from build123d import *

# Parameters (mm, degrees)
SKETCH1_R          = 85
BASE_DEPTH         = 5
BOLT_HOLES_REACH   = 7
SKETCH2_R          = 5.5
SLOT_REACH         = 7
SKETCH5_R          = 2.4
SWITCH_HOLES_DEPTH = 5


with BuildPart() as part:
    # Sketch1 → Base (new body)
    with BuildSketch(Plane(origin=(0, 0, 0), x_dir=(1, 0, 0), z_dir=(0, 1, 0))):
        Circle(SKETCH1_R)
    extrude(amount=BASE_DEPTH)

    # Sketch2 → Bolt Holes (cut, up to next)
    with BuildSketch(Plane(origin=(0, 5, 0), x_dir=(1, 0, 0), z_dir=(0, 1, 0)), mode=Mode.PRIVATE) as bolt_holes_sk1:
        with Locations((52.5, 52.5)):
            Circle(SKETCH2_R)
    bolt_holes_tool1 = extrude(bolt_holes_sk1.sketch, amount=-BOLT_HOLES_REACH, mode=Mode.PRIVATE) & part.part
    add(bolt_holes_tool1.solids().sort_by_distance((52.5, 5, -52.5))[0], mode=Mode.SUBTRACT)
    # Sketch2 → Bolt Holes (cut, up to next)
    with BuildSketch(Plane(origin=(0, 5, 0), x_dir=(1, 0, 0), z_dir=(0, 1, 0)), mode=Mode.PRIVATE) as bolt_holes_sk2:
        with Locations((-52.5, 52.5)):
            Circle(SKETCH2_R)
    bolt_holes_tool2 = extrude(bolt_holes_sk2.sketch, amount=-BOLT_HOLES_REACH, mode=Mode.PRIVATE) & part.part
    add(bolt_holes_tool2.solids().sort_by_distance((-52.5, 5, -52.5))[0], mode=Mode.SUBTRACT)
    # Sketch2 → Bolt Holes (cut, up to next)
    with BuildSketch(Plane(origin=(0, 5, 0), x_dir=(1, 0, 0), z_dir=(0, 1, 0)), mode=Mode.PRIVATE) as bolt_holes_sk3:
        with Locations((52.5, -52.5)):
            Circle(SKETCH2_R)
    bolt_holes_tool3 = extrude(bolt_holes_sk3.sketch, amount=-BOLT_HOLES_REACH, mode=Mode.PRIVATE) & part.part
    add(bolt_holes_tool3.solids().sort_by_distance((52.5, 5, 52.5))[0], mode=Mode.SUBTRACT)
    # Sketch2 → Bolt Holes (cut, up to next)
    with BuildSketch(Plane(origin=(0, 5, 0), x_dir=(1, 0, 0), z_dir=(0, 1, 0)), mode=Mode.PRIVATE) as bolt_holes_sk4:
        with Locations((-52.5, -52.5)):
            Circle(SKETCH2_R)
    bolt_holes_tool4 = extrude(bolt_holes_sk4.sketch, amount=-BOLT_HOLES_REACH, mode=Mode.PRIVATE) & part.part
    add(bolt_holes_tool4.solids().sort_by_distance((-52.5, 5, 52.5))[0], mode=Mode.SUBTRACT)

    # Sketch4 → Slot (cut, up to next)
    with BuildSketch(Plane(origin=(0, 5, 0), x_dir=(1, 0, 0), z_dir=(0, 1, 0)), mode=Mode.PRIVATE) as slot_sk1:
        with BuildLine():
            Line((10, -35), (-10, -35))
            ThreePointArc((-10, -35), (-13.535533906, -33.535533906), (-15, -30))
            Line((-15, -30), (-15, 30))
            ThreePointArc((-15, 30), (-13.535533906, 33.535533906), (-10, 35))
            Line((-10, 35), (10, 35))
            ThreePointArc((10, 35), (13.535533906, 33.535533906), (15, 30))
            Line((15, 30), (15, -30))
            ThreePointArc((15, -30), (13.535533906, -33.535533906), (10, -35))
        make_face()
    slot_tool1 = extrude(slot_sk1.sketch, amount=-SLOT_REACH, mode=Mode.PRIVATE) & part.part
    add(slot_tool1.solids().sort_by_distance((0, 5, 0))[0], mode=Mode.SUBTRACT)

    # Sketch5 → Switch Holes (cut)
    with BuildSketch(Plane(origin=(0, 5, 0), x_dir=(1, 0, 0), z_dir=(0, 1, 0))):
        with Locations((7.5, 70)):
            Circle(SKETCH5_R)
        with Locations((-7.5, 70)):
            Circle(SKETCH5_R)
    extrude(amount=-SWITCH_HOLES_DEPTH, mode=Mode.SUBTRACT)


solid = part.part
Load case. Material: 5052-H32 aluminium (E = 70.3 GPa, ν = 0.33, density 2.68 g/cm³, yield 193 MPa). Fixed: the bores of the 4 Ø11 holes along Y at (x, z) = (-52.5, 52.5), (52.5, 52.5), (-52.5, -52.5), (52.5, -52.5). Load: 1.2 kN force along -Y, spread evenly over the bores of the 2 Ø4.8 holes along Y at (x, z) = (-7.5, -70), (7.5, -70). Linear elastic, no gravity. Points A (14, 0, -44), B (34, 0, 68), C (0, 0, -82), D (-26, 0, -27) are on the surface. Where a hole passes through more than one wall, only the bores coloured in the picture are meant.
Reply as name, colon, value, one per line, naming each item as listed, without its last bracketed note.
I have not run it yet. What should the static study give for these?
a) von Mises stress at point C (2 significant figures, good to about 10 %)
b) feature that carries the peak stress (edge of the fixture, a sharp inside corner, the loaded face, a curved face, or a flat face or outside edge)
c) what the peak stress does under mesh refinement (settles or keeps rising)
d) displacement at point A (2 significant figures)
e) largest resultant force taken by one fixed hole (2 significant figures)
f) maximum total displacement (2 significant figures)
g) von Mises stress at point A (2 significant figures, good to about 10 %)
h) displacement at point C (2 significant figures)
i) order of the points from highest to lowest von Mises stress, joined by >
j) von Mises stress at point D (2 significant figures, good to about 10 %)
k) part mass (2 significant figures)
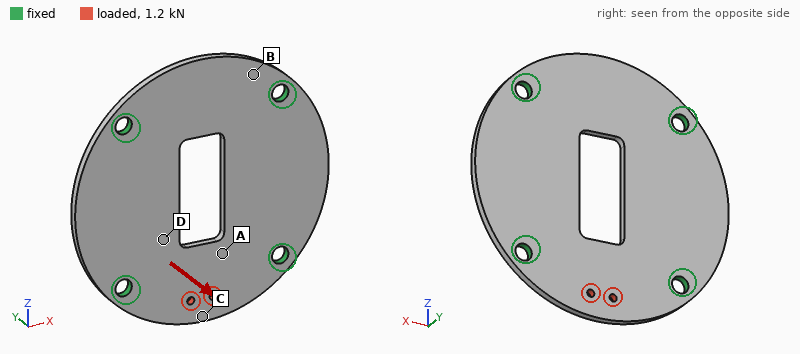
von Mises stress at point C: 73 MPa
feature that carries the peak stress: edge of the fixture
what the peak stress does under mesh refinement: keeps rising
displacement at point A: 0.091 mm
largest resultant force taken by one fixed hole: 640 N
maximum total displacement: 0.40 mm
von Mises stress at point A: 38 MPa
displacement at point C: 0.38 mm
order of the points from highest to lowest von Mises stress, joined by >: C > A > D > B
von Mises stress at point D: 21 MPa
part mass: 270 g
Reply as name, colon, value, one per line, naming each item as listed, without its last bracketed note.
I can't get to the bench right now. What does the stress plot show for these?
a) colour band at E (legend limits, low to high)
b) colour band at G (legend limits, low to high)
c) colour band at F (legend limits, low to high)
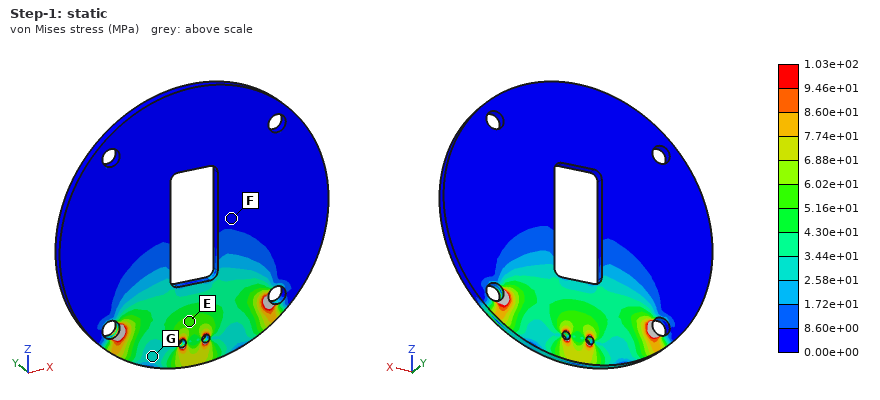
colour band at E: 5.16e+01 to 6.02e+01 MPa
colour band at G: 2.58e+01 to 3.44e+01 MPa
colour band at F: 0.00e+00 to 8.60e+00 MPa
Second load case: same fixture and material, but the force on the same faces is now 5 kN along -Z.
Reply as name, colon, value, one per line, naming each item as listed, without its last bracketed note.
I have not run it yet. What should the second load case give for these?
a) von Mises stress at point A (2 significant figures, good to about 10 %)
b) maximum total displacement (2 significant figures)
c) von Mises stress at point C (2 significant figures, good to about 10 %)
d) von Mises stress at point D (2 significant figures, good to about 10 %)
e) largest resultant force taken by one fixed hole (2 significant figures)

von Mises stress at point A: 22 MPa
maximum total displacement: 24 µm
von Mises stress at point C: 25 MPa
von Mises stress at point D: 12 MPa
largest resultant force taken by one fixed hole: 1.8 kN
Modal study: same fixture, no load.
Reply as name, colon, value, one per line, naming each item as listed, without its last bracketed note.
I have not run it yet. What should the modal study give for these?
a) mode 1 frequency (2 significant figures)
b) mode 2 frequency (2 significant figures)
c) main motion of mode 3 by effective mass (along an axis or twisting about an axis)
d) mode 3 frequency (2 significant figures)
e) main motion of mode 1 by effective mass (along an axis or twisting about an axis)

mode 1 frequency: 2000 Hz
mode 2 frequency: 2100 Hz
main motion of mode 3 by effective mass: twisting about Z
mode 3 frequency: 2200 Hz
main motion of mode 1 by effective mass: along Y
